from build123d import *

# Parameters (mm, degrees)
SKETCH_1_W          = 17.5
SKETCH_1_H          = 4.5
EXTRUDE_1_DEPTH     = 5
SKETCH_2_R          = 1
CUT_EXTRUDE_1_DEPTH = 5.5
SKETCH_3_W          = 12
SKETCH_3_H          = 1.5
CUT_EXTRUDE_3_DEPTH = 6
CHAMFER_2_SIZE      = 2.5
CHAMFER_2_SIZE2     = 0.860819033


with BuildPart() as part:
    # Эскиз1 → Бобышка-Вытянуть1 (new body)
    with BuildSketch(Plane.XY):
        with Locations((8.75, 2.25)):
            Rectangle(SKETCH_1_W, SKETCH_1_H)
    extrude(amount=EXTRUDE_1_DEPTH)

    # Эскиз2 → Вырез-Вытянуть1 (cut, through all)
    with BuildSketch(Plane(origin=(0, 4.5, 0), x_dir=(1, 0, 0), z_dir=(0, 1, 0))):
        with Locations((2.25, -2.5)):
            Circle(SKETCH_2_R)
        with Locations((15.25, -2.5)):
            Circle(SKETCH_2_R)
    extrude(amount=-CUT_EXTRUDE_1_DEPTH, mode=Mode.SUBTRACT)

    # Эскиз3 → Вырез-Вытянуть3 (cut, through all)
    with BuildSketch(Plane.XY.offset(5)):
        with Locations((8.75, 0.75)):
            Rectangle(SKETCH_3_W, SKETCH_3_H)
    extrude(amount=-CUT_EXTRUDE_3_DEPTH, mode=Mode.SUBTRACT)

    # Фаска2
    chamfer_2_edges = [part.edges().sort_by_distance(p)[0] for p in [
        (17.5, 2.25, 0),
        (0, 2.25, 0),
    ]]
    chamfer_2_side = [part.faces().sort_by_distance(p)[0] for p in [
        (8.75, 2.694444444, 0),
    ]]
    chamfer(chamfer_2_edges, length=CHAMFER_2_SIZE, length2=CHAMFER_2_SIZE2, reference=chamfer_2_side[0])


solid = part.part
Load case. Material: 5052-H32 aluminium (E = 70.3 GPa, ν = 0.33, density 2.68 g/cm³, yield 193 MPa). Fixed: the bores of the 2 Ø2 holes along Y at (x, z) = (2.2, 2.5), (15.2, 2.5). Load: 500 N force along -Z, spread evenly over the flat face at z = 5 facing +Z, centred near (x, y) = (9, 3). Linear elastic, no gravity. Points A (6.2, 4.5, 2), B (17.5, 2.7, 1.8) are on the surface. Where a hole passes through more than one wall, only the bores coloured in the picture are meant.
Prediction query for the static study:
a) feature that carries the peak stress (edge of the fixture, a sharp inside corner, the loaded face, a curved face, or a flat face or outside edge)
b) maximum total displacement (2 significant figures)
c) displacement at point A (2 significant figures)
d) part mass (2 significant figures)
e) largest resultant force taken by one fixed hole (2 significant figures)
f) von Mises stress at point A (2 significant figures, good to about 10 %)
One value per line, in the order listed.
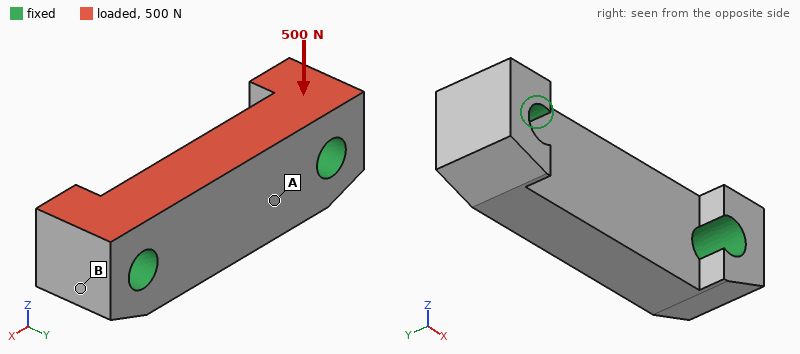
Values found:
edge of the fixture
2.5 µm
1.7 µm
0.72 g
250 N
11 MPa
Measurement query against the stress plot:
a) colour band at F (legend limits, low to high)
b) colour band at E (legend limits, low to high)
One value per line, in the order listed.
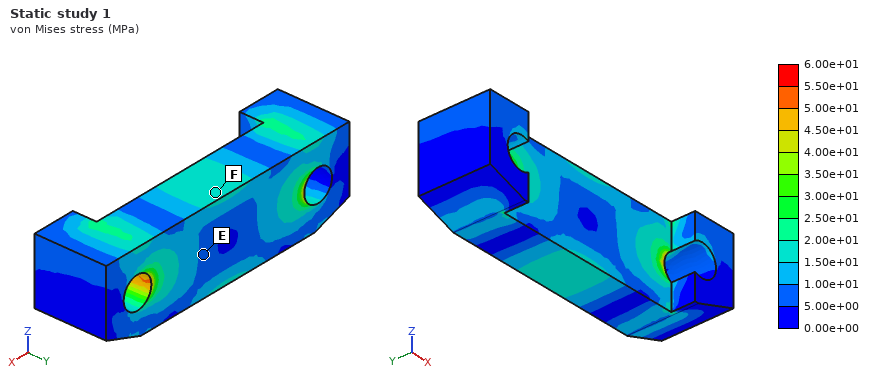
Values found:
1.50e+01 to 2.00e+01 MPa
5.00e+00 to 1.00e+01 MPa
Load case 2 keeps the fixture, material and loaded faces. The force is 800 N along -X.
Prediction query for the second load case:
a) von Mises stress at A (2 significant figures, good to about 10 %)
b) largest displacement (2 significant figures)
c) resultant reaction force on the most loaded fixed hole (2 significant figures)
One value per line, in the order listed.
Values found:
11 MPa
2.5 µm
410 N
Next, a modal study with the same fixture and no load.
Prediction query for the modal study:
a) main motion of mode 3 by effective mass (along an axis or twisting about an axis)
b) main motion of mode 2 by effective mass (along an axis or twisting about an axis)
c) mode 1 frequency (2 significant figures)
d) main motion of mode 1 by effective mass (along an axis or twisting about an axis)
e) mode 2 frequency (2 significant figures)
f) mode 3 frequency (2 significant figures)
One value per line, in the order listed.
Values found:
twisting about X
along Z
81 kHz
along Y
89 kHz
110 kHz
